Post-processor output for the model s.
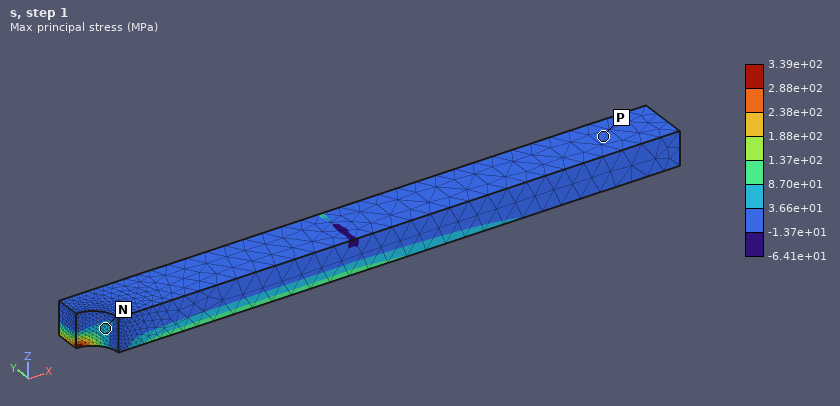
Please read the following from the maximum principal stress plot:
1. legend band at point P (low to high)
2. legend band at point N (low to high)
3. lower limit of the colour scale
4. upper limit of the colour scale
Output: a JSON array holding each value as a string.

["-1.37e+01 to 3.66e+01 MPa", "3.66e+01 to 8.70e+01 MPa", "-6.41e+01 MPa", "3.39e+02 MPa"]
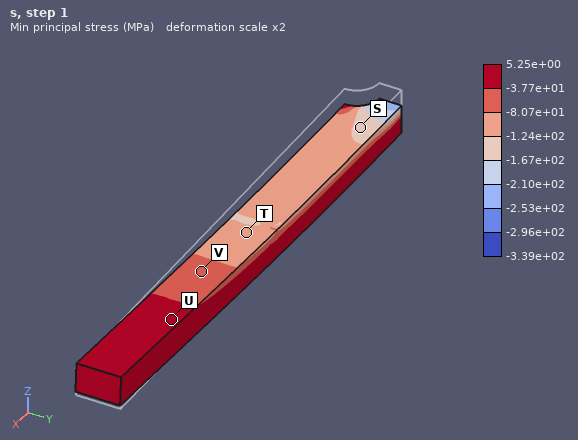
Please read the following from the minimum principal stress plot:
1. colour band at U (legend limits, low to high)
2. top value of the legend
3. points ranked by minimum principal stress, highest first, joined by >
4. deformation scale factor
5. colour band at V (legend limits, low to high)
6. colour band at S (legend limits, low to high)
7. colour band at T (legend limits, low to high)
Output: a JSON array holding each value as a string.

["-3.77e+01 to 5.25e+00 MPa", "5.25e+00 MPa", "U > V > T > S", "2", "-8.07e+01 to -3.77e+01 MPa", "-1.67e+02 to -1.24e+02 MPa", "-1.24e+02 to -8.07e+01 MPa"]
